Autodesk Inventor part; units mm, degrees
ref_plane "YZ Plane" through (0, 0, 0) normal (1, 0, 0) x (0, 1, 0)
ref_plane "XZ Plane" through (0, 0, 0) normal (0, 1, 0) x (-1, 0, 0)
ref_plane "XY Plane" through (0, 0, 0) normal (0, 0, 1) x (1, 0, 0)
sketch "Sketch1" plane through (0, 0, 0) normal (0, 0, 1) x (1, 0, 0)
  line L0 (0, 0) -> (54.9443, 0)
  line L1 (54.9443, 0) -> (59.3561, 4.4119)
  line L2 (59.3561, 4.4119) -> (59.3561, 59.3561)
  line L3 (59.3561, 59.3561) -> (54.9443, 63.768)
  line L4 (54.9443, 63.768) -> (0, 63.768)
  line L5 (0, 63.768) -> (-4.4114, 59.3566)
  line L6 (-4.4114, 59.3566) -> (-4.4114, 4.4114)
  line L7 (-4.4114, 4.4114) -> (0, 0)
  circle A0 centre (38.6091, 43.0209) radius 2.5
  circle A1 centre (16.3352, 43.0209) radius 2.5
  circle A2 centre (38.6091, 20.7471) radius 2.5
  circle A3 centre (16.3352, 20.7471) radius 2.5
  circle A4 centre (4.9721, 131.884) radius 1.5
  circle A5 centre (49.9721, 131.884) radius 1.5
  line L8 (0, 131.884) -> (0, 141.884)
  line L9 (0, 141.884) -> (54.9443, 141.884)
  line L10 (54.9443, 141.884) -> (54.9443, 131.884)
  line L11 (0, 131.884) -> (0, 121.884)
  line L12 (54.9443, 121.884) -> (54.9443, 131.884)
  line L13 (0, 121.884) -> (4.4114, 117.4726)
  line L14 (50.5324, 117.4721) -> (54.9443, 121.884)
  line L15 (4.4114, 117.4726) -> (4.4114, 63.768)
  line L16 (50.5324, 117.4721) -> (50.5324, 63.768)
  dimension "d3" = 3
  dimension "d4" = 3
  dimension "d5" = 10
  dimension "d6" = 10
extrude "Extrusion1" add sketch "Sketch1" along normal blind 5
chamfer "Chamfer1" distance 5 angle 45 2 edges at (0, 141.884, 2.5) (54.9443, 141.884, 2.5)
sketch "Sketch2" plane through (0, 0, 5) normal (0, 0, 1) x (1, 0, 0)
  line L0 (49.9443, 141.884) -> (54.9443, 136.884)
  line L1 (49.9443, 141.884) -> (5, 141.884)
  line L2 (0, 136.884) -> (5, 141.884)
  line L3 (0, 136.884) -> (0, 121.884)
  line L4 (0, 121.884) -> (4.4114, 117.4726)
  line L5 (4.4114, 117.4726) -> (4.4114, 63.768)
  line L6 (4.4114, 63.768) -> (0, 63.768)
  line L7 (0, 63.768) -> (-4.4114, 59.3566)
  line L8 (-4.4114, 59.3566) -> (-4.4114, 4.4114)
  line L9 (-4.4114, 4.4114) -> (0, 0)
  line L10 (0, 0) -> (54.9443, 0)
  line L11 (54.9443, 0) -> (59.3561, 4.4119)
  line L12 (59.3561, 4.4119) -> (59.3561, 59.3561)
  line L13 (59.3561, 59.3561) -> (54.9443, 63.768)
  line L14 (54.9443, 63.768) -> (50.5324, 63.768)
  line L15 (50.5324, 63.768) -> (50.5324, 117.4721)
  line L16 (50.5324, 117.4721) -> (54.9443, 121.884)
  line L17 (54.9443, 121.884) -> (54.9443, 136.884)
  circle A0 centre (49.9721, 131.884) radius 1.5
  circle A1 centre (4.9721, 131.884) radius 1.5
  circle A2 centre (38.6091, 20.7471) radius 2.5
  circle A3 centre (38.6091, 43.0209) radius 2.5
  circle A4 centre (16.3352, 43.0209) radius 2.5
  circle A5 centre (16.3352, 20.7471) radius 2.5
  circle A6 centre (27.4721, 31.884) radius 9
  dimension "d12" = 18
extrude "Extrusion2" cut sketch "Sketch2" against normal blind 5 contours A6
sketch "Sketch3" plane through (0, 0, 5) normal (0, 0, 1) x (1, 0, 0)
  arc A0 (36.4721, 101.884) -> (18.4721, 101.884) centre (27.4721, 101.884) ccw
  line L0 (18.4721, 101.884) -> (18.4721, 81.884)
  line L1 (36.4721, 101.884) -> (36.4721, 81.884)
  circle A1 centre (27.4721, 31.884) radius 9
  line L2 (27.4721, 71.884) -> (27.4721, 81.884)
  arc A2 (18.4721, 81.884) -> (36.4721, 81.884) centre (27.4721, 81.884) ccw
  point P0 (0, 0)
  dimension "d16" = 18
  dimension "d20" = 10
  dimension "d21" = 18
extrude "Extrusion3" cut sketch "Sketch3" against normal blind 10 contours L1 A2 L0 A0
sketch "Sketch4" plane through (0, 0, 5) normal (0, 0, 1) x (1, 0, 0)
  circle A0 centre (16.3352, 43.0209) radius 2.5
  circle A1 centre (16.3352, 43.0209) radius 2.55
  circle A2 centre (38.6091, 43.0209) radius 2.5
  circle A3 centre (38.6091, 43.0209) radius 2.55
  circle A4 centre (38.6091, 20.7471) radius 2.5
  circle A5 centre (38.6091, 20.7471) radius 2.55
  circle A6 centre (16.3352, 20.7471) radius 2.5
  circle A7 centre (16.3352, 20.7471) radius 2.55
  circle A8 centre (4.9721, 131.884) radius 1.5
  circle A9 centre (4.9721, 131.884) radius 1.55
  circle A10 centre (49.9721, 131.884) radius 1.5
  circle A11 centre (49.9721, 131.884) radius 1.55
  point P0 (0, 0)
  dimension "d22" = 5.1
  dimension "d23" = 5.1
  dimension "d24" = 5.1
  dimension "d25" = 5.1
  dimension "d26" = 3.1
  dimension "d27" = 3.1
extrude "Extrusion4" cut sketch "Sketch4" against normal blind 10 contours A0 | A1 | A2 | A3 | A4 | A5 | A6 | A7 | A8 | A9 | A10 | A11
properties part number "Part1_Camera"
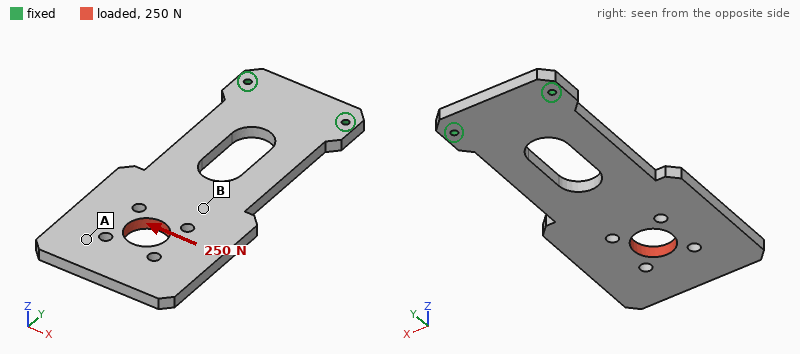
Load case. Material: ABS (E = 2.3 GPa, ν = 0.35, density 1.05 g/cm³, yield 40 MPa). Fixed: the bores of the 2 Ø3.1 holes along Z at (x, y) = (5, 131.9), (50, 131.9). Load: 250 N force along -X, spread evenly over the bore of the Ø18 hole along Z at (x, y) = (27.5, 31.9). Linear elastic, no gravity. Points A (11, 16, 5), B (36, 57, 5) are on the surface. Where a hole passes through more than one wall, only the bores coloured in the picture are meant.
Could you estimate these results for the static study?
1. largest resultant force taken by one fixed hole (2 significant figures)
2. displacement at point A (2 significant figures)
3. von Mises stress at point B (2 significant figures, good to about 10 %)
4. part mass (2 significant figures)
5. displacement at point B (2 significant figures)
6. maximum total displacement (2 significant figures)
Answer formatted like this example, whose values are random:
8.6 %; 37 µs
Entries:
560 N; 1.5 mm; 3.6 MPa; 36 g; 0.96 mm; 1.8 mm
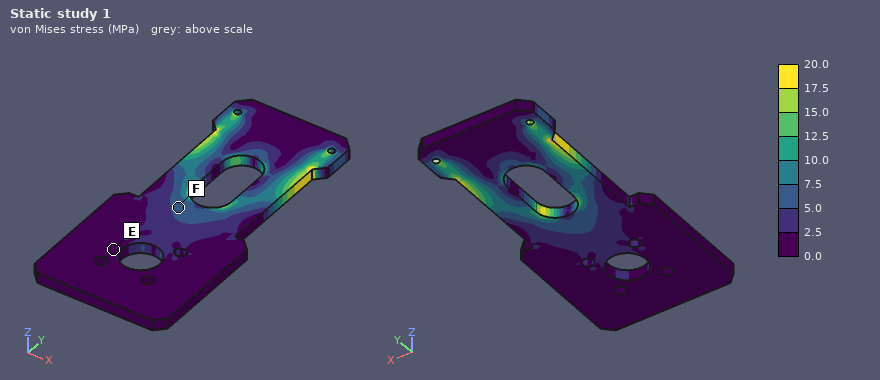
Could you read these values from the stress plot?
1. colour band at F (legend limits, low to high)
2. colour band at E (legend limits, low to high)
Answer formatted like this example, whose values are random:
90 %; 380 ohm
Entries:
5.0 to 7.5 MPa; 0.0 to 2.5 MPa
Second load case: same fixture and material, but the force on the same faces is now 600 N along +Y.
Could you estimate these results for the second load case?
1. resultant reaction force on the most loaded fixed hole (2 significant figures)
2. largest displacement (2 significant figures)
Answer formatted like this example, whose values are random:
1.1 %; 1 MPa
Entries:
310 N; 0.19 mm
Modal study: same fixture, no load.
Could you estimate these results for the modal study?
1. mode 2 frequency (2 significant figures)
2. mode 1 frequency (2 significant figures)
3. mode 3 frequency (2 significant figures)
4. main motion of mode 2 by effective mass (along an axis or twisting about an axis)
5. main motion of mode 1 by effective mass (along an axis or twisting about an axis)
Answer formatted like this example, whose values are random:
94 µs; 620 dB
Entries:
230 Hz; 53 Hz; 390 Hz; twisting about Y; along Z
